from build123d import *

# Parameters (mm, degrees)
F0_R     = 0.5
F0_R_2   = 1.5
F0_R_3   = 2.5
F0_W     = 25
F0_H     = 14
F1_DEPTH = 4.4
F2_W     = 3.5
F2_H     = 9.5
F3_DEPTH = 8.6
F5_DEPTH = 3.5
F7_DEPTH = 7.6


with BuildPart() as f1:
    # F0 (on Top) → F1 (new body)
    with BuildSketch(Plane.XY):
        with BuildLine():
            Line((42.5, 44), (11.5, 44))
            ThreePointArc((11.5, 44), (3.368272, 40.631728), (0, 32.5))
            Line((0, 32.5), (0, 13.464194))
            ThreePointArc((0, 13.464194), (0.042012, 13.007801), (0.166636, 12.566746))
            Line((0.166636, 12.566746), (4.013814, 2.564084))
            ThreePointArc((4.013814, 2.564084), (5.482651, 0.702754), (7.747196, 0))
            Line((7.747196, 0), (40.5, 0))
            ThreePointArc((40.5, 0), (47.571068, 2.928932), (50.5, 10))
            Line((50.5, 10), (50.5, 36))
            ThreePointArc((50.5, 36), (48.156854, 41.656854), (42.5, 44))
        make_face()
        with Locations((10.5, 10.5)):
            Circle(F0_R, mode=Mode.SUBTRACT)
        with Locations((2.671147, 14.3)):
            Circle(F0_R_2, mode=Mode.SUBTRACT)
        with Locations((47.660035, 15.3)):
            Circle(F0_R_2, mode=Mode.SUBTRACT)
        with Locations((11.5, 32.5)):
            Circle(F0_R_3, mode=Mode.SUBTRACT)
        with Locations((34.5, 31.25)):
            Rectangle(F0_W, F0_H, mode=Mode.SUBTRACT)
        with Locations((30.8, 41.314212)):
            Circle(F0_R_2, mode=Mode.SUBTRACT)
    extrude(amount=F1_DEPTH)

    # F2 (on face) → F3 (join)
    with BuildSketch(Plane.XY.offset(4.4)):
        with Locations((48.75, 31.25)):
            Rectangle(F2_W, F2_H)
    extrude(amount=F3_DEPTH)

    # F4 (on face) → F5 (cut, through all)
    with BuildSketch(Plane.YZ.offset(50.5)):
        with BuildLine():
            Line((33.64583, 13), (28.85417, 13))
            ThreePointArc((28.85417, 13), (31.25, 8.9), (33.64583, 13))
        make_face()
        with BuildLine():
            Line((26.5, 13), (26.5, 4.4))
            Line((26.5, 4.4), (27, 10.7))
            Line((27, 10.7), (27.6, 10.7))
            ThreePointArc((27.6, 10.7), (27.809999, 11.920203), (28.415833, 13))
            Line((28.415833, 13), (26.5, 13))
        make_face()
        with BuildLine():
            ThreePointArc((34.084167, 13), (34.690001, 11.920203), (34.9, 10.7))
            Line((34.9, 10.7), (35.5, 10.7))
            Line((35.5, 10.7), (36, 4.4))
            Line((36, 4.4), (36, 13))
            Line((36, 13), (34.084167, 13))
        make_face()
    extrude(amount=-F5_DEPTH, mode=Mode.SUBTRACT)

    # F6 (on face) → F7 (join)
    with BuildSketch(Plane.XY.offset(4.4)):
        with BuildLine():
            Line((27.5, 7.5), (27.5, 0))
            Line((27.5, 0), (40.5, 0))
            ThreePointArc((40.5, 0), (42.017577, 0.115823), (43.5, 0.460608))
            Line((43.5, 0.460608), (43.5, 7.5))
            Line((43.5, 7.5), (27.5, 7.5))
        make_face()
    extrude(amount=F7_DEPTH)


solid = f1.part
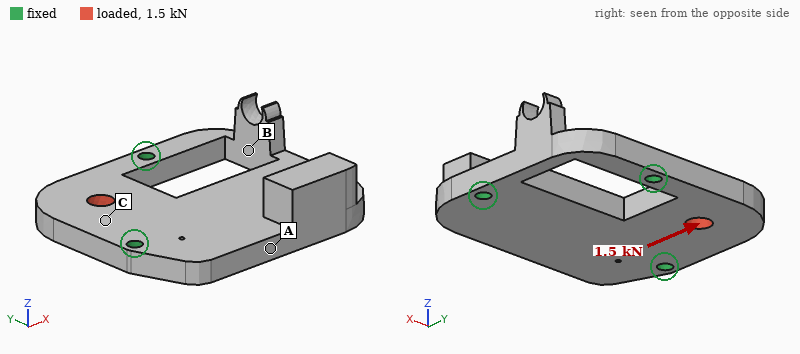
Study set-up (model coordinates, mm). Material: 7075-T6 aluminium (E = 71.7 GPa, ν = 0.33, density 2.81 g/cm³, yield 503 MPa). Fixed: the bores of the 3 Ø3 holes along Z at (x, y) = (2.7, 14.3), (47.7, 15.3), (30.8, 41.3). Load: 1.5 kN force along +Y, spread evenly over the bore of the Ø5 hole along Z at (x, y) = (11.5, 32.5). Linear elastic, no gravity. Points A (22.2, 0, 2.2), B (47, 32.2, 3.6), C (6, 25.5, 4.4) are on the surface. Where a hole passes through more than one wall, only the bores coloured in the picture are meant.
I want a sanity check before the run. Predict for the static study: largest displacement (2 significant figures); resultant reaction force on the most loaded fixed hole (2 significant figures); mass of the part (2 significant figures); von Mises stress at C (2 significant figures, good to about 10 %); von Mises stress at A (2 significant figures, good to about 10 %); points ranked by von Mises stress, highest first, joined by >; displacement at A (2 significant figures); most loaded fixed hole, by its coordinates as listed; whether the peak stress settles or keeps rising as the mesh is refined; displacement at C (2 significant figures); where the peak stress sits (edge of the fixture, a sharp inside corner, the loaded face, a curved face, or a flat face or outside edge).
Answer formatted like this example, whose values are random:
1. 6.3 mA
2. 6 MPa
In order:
1. 8.4 µm
2. 1.2 kN
3. 25 g
4. 20 MPa
5. 11 MPa
6. C > A > B
7. 3.8 µm
8. (2.7, 14.3)
9. keeps rising
10. 4.1 µm
11. edge of the fixture
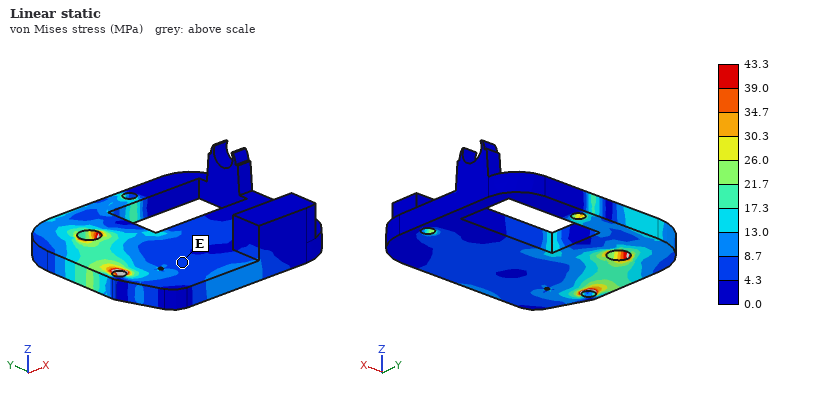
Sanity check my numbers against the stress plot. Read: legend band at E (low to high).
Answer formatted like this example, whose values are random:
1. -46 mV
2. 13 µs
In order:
1. 4.3 to 8.7 MPa
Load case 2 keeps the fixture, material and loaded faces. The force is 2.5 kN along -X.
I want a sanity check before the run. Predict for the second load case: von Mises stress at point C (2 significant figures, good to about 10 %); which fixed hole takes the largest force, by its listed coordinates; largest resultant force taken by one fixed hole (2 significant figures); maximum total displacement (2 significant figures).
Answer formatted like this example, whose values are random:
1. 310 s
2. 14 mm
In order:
1. 21 MPa
2. (30.8, 41.3)
3. 1.2 kN
4. 14 µm
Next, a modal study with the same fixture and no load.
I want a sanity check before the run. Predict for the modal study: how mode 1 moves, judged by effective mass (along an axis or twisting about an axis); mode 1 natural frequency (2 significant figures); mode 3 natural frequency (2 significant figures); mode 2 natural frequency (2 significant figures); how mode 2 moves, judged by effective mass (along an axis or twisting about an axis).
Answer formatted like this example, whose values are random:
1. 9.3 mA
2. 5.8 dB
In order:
1. along Z
2. 6300 Hz
3. 10 kHz
4. 7900 Hz
5. along Z
